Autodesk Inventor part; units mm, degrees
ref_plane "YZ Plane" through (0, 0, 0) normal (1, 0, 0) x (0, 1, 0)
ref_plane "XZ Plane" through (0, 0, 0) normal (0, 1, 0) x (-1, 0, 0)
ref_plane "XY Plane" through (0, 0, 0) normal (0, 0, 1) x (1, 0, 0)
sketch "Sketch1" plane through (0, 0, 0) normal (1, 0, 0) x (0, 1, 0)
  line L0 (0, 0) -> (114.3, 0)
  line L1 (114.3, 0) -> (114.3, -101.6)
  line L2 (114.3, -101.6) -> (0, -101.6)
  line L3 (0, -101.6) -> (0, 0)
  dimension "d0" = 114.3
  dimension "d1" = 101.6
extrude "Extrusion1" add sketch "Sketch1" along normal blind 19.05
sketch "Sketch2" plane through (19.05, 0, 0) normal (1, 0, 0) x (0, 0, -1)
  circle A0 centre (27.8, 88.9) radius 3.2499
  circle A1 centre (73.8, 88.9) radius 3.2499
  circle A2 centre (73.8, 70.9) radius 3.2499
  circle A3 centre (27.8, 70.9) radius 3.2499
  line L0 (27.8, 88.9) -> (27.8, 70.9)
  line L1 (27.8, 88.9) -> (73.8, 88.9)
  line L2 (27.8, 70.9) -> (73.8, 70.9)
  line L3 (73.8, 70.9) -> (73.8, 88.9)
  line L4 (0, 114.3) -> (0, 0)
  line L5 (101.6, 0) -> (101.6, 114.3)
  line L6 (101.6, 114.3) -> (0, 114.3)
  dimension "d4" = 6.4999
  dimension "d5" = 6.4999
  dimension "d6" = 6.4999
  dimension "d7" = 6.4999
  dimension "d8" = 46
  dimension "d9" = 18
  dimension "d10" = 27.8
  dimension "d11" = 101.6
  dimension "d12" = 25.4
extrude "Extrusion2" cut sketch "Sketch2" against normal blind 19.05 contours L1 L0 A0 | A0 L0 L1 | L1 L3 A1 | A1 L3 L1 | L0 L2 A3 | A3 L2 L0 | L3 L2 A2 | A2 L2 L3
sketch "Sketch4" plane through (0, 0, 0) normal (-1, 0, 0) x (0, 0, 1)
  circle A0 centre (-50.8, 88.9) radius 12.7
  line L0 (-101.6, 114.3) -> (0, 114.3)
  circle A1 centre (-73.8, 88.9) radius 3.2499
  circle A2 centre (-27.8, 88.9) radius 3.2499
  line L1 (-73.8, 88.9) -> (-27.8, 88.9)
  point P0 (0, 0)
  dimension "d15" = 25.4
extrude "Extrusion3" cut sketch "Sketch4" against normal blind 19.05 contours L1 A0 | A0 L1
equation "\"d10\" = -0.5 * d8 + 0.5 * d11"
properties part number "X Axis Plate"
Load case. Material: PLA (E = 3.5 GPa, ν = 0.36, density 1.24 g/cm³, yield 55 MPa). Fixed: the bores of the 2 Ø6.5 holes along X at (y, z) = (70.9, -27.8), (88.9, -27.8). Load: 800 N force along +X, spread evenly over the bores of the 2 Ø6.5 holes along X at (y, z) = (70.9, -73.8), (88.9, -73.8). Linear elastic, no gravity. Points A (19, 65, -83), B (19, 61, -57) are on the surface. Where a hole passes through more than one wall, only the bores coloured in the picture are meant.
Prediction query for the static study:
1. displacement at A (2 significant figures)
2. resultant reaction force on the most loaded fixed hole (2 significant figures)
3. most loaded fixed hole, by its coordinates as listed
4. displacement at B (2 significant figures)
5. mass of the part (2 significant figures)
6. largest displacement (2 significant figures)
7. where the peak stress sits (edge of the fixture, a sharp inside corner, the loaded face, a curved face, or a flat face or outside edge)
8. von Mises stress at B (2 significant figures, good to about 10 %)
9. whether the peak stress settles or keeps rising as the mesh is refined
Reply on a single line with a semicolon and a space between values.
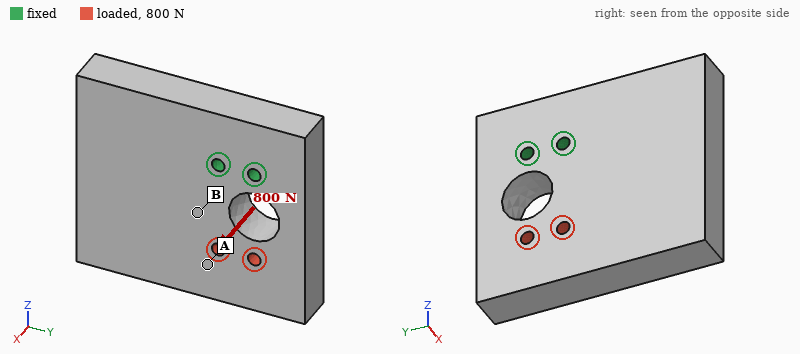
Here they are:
0.40 mm; 460 N; (70.9, -27.8); 0.18 mm; 260 g; 0.59 mm; edge of the fixture; 3.5 MPa; keeps rising
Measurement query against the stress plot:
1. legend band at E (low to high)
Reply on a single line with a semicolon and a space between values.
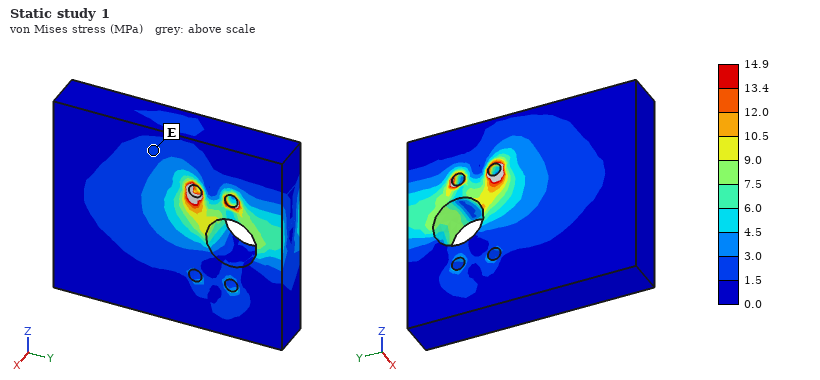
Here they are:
1.5 to 3.0 MPa
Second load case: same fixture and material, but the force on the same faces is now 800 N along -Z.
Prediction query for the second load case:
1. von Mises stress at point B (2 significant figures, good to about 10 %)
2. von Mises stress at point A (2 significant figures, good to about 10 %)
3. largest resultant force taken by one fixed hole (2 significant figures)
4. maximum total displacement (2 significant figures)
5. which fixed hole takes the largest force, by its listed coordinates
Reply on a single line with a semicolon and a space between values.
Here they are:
0.69 MPa; 0.86 MPa; 450 N; 27 µm; (70.9, -27.8)
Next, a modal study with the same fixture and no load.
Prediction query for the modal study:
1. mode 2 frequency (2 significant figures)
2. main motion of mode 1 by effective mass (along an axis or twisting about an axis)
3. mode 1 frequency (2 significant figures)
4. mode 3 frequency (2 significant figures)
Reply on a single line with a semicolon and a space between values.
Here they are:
720 Hz; along X; 530 Hz; 780 Hz
